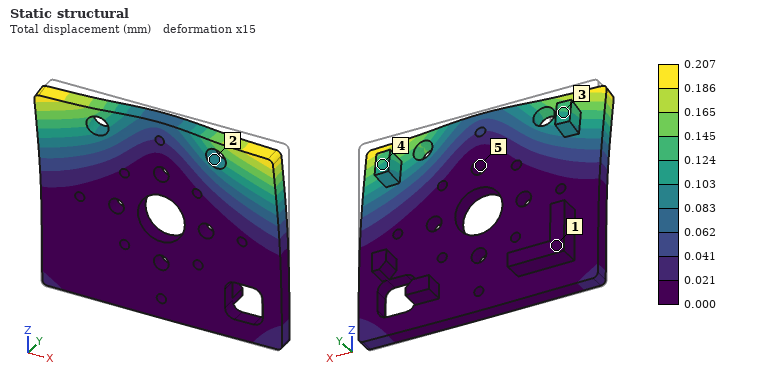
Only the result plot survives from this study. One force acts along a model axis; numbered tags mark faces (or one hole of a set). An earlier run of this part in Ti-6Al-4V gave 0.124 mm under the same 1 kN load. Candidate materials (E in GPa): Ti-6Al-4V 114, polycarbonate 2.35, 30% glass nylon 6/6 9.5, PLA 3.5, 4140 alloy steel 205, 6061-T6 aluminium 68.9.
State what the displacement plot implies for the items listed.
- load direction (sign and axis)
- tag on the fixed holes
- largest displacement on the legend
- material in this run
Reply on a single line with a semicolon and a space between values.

-Y; 5; 0.207 mm; 6061-T6 aluminium
